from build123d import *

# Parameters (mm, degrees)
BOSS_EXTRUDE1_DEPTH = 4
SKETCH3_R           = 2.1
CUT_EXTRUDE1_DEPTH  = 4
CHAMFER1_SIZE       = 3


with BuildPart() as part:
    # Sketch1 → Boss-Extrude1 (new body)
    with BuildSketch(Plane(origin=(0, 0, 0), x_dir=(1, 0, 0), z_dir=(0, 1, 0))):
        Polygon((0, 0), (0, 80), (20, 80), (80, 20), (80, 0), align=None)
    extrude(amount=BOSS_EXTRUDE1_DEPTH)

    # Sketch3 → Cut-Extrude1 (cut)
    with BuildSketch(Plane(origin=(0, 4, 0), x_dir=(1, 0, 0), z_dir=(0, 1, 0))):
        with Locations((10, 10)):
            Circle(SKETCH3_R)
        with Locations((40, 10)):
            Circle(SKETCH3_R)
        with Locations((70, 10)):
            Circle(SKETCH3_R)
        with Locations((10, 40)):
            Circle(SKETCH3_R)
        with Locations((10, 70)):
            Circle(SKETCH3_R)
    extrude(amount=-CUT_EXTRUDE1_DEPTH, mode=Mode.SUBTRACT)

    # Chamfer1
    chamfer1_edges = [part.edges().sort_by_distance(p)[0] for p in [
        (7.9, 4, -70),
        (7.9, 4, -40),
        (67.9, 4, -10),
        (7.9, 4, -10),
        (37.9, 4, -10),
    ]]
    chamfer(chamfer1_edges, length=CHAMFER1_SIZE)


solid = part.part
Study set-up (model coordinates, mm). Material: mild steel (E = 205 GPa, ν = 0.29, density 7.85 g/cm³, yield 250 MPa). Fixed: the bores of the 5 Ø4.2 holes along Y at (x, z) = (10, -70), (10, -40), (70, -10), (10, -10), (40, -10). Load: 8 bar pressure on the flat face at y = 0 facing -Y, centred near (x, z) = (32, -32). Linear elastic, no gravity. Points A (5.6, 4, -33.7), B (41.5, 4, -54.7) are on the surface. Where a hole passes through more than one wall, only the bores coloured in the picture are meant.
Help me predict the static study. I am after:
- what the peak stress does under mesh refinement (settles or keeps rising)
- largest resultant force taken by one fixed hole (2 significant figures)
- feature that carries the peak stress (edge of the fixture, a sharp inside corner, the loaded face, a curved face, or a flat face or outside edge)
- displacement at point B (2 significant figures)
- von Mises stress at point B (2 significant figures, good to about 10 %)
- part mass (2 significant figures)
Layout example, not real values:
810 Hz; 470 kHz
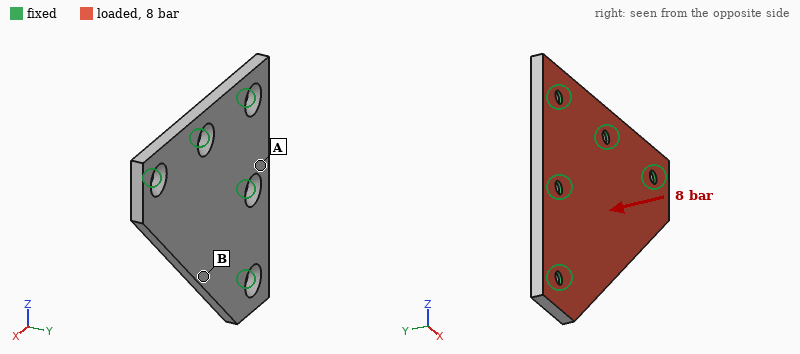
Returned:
keeps rising; 1.3 kN; edge of the fixture; 0.11 mm; 70 MPa; 140 g
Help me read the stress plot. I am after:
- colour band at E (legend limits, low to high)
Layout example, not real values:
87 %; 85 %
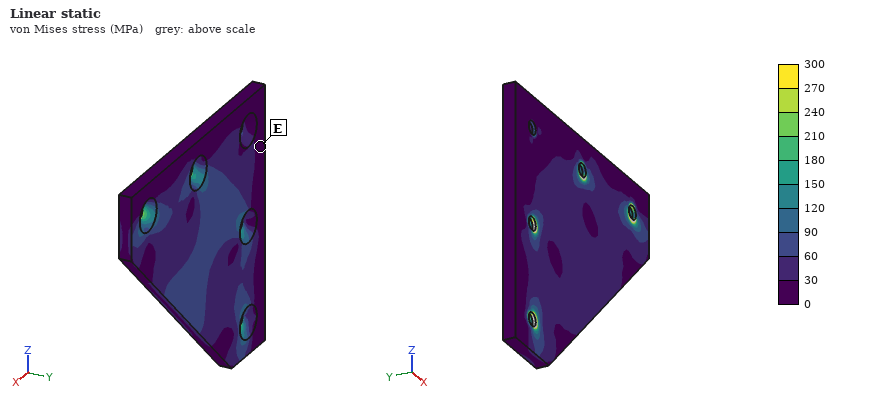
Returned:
0 to 30 MPa
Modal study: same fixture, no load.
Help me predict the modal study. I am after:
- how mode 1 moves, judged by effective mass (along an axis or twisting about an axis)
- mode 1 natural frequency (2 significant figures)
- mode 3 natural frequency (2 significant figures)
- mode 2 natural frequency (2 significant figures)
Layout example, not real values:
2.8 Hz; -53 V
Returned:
along Y; 2900 Hz; 9900 Hz; 6400 Hz
